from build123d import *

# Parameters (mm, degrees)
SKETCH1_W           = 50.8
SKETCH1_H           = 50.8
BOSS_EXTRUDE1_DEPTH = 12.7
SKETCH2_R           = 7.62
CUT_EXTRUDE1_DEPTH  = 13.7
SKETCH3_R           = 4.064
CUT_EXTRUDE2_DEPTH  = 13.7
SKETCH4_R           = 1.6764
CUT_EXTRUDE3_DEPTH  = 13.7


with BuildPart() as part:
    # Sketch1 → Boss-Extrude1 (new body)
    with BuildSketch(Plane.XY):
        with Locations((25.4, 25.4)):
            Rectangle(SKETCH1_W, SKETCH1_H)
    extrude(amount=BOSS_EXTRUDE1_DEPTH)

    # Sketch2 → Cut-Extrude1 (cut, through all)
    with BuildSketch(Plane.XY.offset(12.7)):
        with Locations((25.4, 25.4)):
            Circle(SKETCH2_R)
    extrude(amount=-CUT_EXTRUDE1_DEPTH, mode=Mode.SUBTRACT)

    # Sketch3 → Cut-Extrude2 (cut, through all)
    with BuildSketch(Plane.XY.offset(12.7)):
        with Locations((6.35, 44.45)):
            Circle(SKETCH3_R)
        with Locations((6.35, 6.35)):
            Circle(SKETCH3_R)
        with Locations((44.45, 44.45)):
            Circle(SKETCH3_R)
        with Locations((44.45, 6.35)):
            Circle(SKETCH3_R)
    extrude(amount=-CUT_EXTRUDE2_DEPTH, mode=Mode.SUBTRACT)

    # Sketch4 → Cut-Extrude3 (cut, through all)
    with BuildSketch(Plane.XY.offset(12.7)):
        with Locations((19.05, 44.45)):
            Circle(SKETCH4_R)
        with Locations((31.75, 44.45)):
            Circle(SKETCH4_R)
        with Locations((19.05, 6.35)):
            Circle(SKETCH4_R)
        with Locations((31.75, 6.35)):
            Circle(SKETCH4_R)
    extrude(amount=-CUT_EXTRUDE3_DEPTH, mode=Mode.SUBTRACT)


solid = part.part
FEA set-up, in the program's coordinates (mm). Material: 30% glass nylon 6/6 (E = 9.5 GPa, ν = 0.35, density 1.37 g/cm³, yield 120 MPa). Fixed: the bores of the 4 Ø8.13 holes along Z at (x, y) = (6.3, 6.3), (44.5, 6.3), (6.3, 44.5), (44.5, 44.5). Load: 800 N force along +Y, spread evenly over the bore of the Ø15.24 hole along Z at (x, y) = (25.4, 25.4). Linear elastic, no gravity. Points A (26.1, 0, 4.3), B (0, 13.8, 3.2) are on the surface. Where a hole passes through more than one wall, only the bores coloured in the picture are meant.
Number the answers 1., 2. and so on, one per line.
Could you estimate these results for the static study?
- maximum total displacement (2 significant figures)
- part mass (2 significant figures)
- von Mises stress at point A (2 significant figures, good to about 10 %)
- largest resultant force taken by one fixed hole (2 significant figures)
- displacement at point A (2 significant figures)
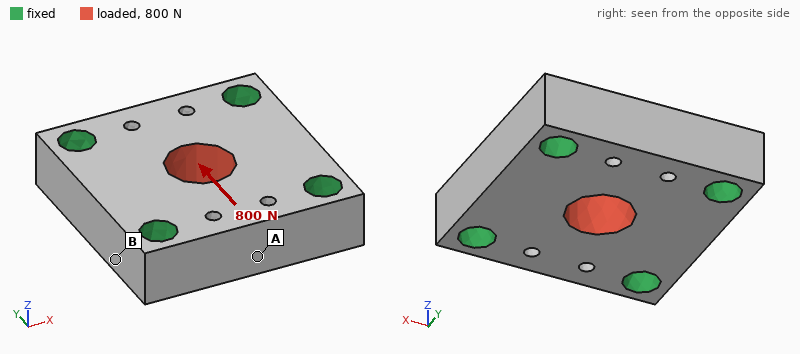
1. 3.6 µm
2. 38 g
3. 0.99 MPa
4. 220 N
5. 2.4 µm
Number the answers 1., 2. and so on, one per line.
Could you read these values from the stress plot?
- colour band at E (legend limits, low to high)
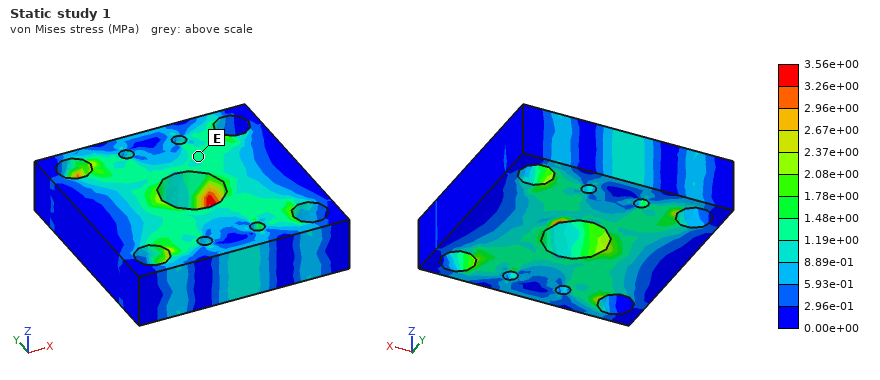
1. 1.19e+00 to 1.48e+00 MPa
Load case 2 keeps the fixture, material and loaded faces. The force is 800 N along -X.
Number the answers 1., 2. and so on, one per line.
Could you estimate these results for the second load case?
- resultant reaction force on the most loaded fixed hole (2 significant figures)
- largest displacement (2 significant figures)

1. 220 N
2. 3.5 µm
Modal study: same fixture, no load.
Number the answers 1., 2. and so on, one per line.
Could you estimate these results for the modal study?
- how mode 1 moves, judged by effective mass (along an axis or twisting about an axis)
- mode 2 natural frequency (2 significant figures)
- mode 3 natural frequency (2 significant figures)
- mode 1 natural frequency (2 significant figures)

1. along Z
2. 19 kHz
3. 19 kHz
4. 14 kHz
